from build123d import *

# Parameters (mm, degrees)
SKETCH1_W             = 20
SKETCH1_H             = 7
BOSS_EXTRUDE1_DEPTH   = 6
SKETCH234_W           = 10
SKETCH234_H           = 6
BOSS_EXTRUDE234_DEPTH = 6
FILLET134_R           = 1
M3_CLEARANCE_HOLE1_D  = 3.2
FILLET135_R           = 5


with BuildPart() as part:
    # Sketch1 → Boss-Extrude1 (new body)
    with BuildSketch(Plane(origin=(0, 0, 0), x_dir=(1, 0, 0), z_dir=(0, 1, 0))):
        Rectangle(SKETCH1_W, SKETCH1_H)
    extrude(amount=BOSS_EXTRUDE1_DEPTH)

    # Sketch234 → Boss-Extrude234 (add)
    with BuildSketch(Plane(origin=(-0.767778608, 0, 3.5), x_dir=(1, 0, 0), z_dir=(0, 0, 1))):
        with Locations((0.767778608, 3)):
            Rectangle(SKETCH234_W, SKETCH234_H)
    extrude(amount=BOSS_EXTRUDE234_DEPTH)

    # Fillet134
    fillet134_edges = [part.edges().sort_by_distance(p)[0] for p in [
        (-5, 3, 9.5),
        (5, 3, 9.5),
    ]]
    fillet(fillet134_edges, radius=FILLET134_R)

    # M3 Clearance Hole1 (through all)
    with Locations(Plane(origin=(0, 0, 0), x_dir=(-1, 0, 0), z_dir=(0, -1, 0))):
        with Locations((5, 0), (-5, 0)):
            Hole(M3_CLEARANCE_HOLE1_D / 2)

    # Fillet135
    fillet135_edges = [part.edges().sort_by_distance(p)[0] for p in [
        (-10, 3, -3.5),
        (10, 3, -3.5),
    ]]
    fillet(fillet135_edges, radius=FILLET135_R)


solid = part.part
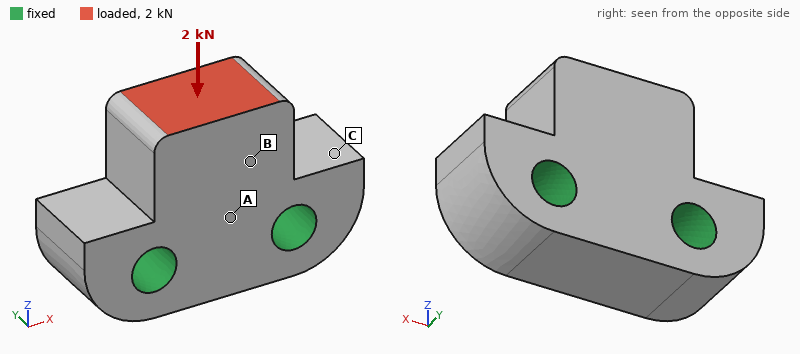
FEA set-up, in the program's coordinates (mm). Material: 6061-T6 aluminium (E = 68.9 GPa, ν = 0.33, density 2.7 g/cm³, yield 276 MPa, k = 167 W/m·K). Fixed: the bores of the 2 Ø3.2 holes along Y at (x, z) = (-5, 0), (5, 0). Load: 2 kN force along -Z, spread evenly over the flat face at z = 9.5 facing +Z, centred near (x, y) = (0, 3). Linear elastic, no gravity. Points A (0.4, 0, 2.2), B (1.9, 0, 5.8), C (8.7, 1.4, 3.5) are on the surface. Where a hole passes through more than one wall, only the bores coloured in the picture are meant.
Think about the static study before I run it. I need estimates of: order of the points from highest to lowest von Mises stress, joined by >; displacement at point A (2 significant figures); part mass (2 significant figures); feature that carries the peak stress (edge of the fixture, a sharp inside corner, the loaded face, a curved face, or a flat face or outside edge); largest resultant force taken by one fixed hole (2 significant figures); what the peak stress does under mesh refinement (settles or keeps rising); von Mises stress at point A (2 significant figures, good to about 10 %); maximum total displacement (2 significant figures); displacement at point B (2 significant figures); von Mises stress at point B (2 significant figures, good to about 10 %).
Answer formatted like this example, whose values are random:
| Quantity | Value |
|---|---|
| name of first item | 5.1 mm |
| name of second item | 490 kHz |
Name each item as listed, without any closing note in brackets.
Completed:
| Quantity | Value |
|---|---|
| order of the points from highest to lowest von Mises stress, joined by > | B > A > C |
| displacement at point A | 1.8 µm |
| part mass | 2.8 g |
| feature that carries the peak stress | edge of the fixture |
| largest resultant force taken by one fixed hole | 1.1 kN |
| what the peak stress does under mesh refinement | keeps rising |
| von Mises stress at point A | 16 MPa |
| maximum total displacement | 5.2 µm |
| displacement at point B | 2.9 µm |
| von Mises stress at point B | 37 MPa |
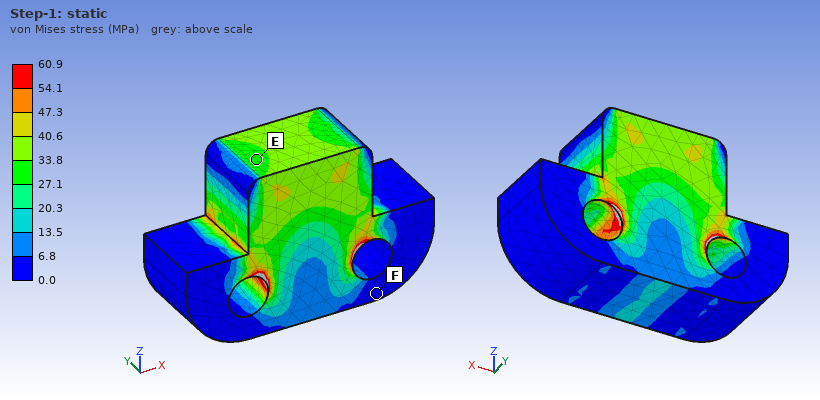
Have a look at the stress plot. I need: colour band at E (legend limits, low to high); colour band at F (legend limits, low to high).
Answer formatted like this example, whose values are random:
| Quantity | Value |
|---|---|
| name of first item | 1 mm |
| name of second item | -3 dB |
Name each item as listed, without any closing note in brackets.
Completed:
| Quantity | Value |
|---|---|
| colour band at E | 27.1 to 33.8 MPa |
| colour band at F | 0.0 to 6.8 MPa |
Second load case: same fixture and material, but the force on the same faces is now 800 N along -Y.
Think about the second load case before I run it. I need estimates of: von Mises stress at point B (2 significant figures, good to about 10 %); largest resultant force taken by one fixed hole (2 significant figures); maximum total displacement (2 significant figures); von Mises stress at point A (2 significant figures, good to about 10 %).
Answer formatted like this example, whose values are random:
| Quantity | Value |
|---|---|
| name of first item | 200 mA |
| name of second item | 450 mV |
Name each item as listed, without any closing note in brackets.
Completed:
| Quantity | Value |
|---|---|
| von Mises stress at point B | 49 MPa |
| largest resultant force taken by one fixed hole | 400 N |
| maximum total displacement | 23 µm |
| von Mises stress at point A | 51 MPa |
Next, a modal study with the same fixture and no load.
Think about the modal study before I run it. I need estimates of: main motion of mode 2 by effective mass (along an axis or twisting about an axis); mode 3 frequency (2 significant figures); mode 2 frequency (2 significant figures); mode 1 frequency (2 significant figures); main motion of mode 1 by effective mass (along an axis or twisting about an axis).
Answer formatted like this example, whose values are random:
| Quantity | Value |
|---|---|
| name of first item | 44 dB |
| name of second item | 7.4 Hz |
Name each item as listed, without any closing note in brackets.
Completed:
| Quantity | Value |
|---|---|
| main motion of mode 2 by effective mass | along X |
| mode 3 frequency | 86 kHz |
| mode 2 frequency | 80 kHz |
| mode 1 frequency | 48 kHz |
| main motion of mode 1 by effective mass | along Y |
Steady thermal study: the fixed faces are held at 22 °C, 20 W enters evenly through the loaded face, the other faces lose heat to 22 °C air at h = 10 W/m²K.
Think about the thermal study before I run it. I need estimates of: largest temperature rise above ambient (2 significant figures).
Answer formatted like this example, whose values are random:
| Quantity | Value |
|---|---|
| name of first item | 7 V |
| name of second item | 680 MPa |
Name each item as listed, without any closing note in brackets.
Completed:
| Quantity | Value |
|---|---|
| largest temperature rise above ambient | 18 K |
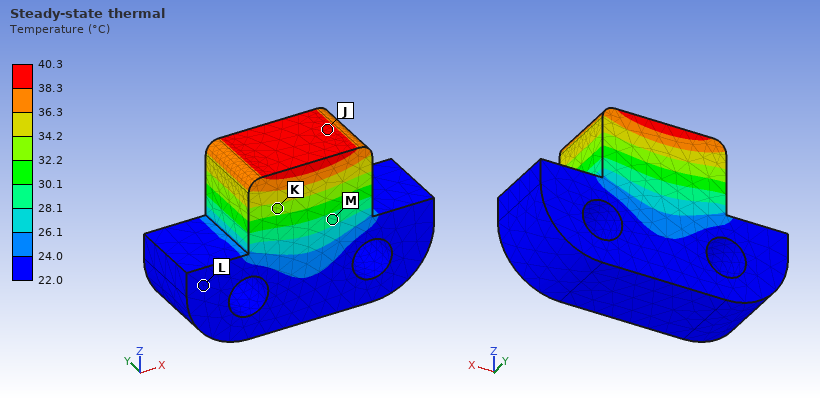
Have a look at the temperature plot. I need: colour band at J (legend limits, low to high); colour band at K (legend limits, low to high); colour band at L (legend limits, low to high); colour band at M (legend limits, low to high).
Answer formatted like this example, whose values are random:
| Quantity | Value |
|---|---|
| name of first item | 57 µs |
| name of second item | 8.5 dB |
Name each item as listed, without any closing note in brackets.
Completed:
| Quantity | Value |
|---|---|
| colour band at J | 38.3 to 40.3 °C |
| colour band at K | 32.2 to 34.2 °C |
| colour band at L | 22.0 to 24.0 °C |
| colour band at M | 28.1 to 30.1 °C |
